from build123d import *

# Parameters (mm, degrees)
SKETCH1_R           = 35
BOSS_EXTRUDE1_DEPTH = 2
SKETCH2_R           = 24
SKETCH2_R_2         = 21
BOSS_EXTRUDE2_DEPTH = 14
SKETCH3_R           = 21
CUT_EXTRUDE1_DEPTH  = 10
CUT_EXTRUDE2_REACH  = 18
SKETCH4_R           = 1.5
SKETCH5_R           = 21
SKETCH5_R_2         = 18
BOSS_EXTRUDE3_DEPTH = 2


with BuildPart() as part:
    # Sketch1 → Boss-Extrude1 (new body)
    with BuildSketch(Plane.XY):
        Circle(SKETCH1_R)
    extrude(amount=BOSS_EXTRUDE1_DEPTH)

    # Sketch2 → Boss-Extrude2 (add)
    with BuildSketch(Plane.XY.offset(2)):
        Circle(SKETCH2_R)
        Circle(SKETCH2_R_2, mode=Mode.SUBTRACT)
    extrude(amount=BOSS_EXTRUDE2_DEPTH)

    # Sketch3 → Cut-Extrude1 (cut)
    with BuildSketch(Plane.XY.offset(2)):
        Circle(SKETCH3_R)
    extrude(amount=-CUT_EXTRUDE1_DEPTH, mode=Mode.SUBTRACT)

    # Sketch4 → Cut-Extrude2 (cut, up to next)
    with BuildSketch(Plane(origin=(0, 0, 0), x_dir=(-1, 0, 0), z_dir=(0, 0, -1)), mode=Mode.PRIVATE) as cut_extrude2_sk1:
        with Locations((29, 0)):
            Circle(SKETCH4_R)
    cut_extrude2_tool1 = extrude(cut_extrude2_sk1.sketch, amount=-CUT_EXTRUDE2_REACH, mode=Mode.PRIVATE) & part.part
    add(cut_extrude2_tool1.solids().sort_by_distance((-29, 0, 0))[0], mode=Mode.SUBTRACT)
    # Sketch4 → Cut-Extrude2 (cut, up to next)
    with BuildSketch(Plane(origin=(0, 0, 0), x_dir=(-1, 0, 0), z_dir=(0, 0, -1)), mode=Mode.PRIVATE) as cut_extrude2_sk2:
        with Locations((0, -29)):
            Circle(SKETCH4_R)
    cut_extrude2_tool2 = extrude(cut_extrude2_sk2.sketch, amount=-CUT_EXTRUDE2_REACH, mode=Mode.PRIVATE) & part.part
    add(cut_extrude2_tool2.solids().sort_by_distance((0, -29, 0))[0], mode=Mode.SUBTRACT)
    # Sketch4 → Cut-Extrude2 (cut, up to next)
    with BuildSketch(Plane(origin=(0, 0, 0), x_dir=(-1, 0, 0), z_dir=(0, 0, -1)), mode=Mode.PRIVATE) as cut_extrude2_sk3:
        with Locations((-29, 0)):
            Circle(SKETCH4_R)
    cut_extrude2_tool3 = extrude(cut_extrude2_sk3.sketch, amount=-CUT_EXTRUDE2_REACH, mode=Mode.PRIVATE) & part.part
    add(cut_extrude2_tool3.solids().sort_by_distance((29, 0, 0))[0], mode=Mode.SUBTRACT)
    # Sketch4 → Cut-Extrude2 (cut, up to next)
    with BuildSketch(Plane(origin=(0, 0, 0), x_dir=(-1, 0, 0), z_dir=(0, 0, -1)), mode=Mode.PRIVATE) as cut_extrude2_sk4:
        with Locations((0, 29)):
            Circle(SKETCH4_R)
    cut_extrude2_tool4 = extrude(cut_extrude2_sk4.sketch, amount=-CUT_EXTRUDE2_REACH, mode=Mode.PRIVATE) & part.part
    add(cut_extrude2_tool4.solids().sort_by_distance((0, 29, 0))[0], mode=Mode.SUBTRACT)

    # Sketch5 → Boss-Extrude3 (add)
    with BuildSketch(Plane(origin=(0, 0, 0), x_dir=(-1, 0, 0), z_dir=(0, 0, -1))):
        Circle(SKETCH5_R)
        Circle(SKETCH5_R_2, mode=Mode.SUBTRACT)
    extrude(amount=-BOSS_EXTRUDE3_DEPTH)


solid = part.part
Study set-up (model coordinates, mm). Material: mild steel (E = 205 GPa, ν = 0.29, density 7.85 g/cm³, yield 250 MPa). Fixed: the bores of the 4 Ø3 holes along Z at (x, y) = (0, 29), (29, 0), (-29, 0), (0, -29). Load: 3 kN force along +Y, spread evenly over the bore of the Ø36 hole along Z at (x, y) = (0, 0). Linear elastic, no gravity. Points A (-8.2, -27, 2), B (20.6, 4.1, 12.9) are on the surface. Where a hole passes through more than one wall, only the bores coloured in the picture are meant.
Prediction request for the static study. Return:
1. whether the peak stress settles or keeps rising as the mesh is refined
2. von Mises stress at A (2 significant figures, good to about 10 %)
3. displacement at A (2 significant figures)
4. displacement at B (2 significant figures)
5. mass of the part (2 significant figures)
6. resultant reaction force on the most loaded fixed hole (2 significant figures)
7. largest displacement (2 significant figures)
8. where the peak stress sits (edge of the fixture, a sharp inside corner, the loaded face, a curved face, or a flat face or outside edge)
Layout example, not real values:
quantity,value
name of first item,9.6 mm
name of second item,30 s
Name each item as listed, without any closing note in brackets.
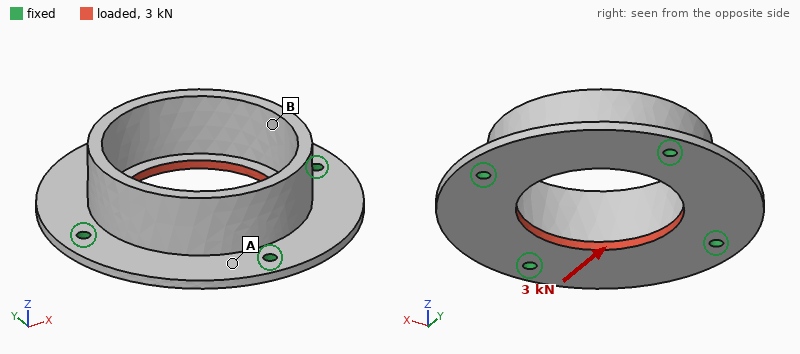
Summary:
quantity,value
whether the peak stress settles or keeps rising as the mesh is refined,keeps rising
von Mises stress at A,12 MPa
displacement at A,1.4 µm
displacement at B,1.6 µm
mass of the part,91 g
resultant reaction force on the most loaded fixed hole,790 N
largest displacement,2.9 µm
where the peak stress sits,edge of the fixture
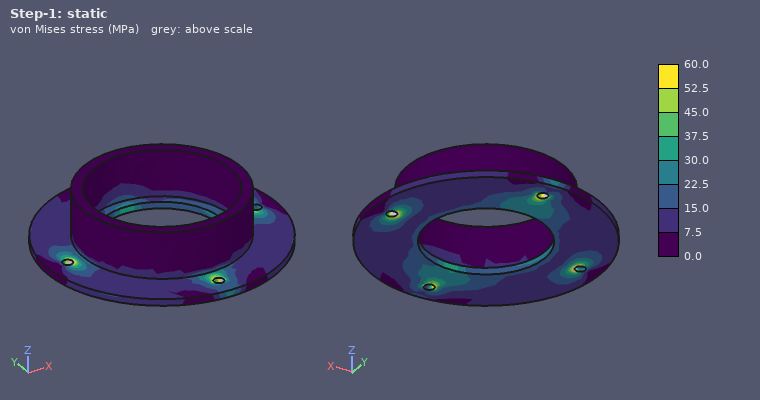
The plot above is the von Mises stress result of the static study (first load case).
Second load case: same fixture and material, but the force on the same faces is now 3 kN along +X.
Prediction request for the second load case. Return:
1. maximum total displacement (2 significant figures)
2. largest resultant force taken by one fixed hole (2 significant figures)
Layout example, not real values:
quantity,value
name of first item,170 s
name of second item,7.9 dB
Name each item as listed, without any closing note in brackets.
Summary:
quantity,value
maximum total displacement,2.9 µm
largest resultant force taken by one fixed hole,790 N
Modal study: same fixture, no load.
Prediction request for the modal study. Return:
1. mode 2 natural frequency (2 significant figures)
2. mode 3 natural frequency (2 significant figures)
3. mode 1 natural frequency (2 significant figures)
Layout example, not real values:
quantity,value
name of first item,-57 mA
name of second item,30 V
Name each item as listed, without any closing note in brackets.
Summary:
quantity,value
mode 2 natural frequency,7700 Hz
mode 3 natural frequency,7700 Hz
mode 1 natural frequency,5800 Hz
